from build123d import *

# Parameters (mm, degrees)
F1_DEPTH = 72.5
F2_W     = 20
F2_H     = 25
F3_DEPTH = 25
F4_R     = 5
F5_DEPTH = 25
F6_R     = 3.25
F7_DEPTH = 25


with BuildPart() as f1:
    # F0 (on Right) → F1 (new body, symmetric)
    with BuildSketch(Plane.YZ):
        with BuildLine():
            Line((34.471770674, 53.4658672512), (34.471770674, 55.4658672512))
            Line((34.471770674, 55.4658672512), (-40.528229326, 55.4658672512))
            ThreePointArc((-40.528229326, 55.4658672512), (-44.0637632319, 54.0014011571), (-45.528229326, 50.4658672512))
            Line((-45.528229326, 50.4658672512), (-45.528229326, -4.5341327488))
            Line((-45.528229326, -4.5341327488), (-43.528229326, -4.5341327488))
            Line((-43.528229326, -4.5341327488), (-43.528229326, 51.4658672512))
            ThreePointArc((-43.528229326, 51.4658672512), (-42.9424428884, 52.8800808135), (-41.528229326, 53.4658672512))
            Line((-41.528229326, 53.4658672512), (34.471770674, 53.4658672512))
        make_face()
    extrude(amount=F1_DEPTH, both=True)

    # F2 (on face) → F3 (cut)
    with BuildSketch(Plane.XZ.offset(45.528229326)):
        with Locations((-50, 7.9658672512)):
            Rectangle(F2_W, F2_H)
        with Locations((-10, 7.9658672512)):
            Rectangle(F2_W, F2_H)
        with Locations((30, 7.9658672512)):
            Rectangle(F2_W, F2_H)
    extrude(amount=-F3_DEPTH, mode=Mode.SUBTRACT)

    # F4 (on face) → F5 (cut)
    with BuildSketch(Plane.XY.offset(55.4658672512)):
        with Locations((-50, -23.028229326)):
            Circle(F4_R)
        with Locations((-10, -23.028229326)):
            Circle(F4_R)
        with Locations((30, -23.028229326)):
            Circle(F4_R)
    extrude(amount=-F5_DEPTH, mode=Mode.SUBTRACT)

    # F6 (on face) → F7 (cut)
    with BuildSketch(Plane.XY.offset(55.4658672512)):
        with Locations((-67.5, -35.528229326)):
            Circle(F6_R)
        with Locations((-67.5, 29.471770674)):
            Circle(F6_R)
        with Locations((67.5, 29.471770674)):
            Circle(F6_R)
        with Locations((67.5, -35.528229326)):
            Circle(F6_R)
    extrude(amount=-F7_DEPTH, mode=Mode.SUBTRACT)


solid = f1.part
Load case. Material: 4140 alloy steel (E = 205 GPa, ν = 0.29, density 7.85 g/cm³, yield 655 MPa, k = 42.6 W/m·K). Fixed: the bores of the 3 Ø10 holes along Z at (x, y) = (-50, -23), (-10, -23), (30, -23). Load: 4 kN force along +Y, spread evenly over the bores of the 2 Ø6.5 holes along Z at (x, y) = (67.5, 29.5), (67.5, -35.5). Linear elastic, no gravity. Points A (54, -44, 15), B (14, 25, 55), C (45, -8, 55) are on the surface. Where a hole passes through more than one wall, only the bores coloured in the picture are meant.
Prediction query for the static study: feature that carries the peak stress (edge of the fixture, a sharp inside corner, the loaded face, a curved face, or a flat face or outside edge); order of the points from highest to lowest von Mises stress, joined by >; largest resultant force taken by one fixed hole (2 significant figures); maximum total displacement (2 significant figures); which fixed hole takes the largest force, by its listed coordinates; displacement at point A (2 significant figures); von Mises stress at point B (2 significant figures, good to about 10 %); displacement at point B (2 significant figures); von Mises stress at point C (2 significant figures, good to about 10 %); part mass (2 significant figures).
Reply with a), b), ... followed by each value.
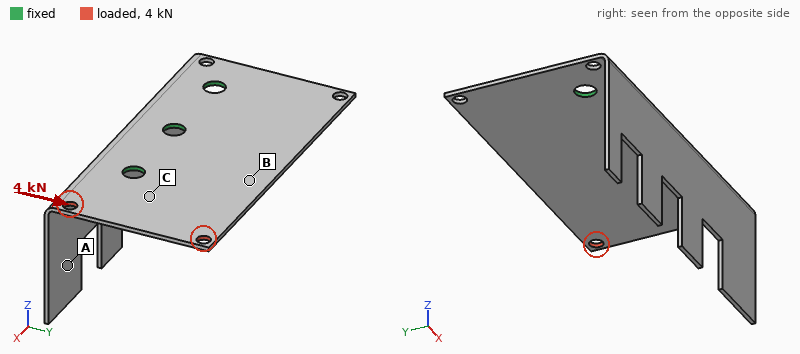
a) the loaded face
b) C > B > A
c) 5.7 kN
d) 55 µm
e) (30, -23)
f) 25 µm
g) 37 MPa
h) 14 µm
i) 69 MPa
j) 280 g
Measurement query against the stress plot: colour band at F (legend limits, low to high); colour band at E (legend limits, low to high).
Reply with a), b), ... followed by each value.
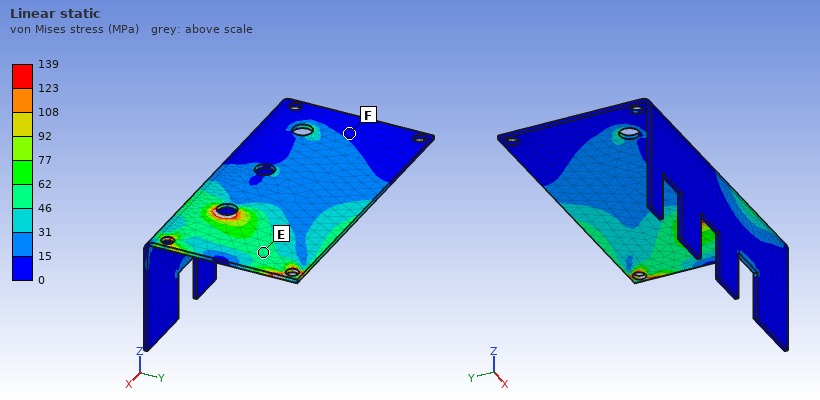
a) 0 to 15 MPa
b) 46 to 62 MPa
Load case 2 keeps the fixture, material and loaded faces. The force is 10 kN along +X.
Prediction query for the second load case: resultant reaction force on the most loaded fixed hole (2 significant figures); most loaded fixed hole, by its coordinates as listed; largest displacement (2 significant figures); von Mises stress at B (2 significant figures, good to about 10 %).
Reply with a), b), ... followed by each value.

a) 6.3 kN
b) (30, -23)
c) 85 µm
d) 66 MPa
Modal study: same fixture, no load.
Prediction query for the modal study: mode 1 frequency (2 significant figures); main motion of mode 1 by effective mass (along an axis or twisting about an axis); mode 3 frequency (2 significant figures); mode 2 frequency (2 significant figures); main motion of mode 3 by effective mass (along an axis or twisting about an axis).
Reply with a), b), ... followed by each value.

a) 360 Hz
b) along Y
c) 530 Hz
d) 470 Hz
e) along Z
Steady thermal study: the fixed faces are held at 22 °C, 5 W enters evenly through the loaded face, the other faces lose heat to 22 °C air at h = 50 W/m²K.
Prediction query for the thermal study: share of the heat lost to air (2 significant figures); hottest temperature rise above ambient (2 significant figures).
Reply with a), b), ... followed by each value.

a) 80 %
b) 38 K
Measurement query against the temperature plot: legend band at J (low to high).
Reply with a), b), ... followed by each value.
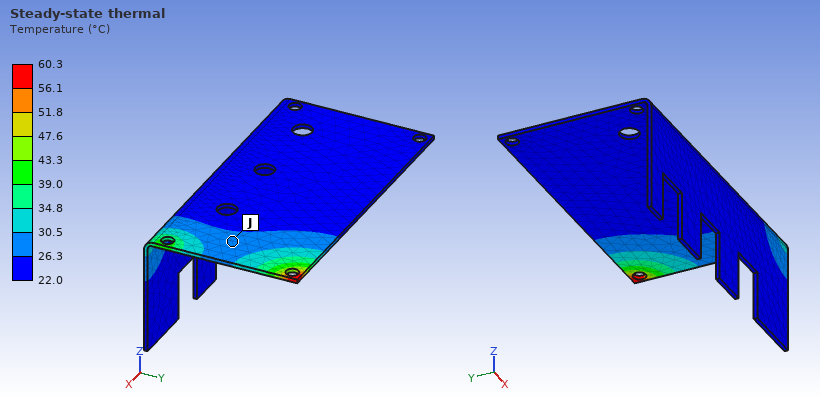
a) 26.3 to 30.5 °C
